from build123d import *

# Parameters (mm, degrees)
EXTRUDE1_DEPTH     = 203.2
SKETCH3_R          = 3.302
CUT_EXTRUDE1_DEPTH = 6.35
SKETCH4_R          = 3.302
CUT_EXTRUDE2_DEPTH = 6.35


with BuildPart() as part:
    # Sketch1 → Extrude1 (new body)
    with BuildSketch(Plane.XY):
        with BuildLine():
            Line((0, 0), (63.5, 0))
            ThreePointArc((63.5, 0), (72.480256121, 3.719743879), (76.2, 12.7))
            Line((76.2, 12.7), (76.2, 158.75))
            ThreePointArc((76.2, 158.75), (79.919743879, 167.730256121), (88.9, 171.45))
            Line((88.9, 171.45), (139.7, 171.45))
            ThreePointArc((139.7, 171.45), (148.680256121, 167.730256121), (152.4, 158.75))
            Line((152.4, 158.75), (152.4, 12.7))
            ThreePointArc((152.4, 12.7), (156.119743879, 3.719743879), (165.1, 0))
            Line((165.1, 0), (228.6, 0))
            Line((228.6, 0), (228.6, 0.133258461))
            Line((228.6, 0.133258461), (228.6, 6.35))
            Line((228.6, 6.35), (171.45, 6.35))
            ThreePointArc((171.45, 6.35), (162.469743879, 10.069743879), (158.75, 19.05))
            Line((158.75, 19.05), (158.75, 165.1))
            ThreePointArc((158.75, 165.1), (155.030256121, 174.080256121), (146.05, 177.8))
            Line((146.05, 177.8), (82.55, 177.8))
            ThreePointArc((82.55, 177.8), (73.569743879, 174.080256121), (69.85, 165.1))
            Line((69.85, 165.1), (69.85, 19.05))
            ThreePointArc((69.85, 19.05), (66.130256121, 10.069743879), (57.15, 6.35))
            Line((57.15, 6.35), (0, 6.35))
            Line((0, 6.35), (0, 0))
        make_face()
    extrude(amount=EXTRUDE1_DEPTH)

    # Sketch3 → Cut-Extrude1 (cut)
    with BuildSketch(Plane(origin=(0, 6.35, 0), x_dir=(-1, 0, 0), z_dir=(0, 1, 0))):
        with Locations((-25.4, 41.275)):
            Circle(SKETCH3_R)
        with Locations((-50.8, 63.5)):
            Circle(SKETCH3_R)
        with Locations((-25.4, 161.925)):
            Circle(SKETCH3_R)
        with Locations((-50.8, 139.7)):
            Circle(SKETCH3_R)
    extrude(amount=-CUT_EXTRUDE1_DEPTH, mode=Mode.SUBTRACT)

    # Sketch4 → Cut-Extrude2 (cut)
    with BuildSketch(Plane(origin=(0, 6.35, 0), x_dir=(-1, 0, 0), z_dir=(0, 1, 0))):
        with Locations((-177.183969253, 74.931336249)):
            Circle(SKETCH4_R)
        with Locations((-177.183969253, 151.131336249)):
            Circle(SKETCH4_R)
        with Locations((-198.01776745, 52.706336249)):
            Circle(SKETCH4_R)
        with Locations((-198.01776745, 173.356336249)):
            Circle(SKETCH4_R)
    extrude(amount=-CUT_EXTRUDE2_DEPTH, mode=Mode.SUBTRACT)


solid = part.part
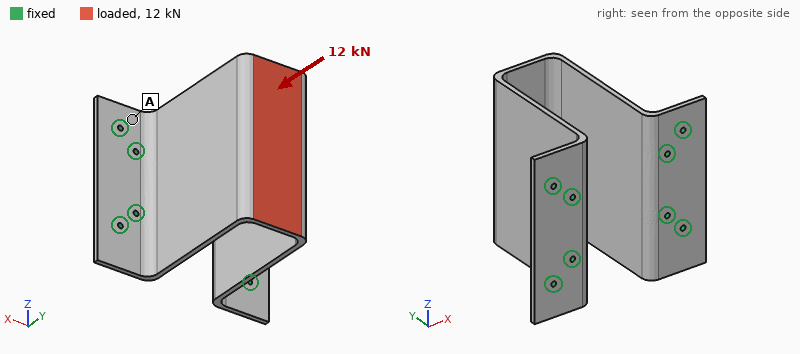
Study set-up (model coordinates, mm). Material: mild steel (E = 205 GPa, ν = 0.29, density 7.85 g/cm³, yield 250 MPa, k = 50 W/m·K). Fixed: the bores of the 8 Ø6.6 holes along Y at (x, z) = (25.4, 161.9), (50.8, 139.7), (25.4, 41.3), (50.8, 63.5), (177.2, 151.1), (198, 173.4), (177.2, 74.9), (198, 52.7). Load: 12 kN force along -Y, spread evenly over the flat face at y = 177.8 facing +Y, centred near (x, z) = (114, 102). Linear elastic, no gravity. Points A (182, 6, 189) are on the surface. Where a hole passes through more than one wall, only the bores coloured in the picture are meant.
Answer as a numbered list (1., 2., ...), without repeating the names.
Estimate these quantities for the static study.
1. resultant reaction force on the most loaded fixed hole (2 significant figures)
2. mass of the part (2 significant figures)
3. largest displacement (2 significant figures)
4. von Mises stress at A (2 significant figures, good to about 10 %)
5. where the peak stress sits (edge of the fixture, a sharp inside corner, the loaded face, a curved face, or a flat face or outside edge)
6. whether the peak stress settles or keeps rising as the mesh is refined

1. 3.7 kN
2. 5.8 kg
3. 0.10 mm
4. 11 MPa
5. edge of the fixture
6. keeps rising
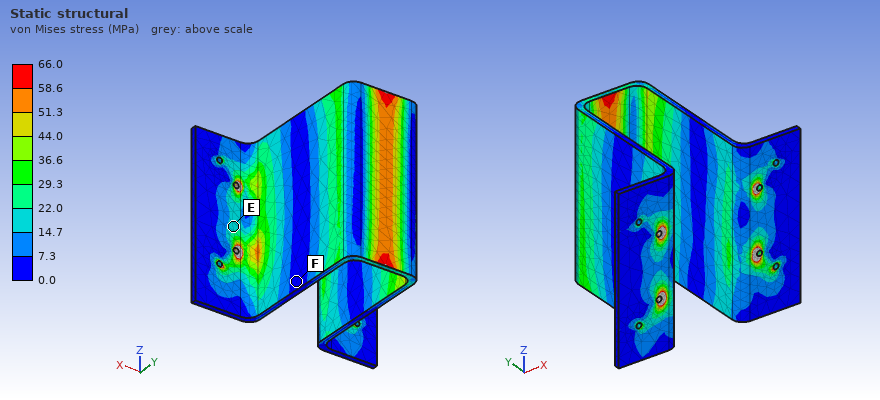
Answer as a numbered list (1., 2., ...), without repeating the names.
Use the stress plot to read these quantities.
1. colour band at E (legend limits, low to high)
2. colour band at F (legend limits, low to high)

1. 14.7 to 22.0 MPa
2. 0.0 to 7.3 MPa
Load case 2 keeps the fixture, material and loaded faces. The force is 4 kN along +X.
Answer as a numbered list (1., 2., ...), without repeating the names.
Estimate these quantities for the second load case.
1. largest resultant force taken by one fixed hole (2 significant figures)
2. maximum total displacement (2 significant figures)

1. 1.5 kN
2. 0.90 mm
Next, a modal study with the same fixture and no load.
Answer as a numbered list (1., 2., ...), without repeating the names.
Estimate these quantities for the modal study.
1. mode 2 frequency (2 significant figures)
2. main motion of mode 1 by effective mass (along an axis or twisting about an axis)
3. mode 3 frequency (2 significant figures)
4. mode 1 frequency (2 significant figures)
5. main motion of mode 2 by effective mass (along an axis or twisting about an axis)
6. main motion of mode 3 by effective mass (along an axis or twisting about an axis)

1. 400 Hz
2. along X
3. 520 Hz
4. 220 Hz
5. twisting about Y
6. along Z
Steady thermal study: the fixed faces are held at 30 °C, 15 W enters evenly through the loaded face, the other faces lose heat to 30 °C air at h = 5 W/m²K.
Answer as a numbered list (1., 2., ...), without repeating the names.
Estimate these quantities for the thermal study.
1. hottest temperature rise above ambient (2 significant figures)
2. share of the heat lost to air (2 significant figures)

1. 17 K
2. 48 %
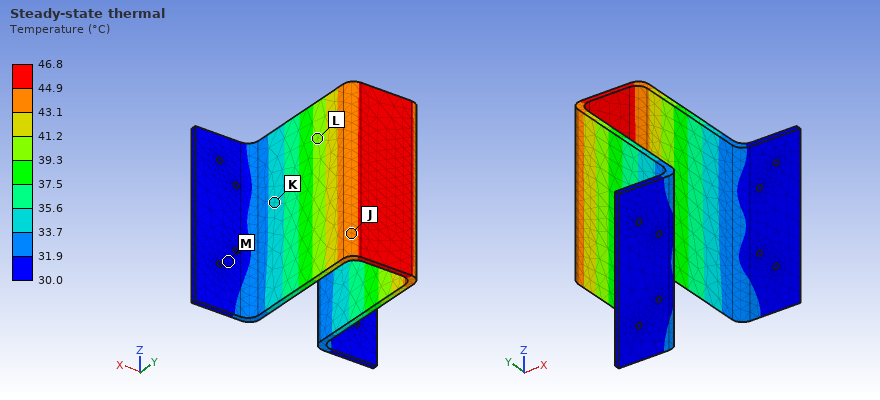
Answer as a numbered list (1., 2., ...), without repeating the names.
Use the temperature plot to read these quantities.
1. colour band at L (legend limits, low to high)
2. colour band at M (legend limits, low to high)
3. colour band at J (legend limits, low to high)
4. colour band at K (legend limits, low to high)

1. 39.3 to 41.2 °C
2. 30.0 to 31.9 °C
3. 43.1 to 44.9 °C
4. 33.7 to 35.6 °C
